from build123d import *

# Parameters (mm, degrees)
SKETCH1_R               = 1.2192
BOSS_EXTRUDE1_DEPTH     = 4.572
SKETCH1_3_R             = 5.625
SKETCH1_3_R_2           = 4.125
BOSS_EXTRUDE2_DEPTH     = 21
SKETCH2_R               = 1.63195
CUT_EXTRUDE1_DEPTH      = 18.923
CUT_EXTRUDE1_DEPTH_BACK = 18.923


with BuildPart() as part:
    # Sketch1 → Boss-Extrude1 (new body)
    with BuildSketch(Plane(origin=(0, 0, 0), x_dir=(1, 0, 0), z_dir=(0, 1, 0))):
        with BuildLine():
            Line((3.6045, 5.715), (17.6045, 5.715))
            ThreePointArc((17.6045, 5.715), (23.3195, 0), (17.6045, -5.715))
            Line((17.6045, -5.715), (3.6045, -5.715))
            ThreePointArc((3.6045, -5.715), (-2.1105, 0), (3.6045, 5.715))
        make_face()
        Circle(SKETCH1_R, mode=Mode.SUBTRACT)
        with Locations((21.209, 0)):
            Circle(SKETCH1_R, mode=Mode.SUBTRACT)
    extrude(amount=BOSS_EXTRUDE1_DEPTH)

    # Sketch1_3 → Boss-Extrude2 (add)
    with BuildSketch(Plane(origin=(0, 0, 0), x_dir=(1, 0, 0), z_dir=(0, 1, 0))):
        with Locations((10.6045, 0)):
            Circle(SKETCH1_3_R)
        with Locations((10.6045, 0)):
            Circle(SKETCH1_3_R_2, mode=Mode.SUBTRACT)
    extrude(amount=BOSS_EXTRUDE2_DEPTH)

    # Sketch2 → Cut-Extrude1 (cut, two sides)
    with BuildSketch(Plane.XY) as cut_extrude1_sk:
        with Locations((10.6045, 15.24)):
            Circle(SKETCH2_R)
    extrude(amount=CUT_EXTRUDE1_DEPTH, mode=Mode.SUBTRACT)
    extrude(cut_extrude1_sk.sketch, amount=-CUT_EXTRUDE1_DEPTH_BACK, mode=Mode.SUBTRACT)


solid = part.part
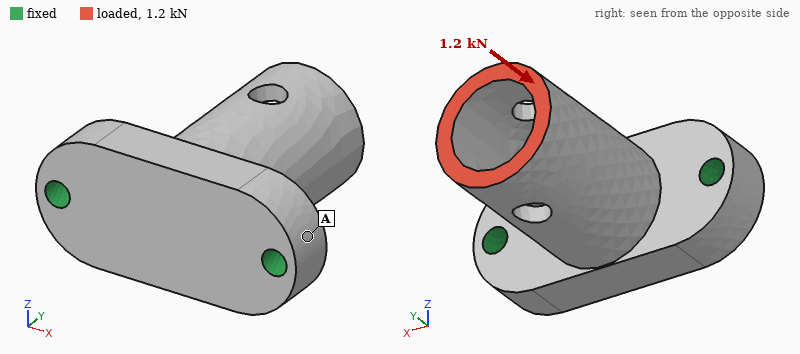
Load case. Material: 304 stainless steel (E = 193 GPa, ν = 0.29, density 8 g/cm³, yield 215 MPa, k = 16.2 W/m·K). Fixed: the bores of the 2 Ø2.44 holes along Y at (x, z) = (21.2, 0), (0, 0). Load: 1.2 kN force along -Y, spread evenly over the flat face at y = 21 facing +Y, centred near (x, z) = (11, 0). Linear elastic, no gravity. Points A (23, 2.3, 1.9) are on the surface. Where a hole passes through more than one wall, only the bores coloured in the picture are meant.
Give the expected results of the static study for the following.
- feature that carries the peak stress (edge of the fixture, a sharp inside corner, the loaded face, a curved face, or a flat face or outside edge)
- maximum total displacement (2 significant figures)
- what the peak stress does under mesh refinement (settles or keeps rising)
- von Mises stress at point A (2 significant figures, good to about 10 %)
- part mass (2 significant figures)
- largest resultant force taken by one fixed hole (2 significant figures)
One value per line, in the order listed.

edge of the fixture
6.1 µm
keeps rising
18 MPa
15 g
610 N
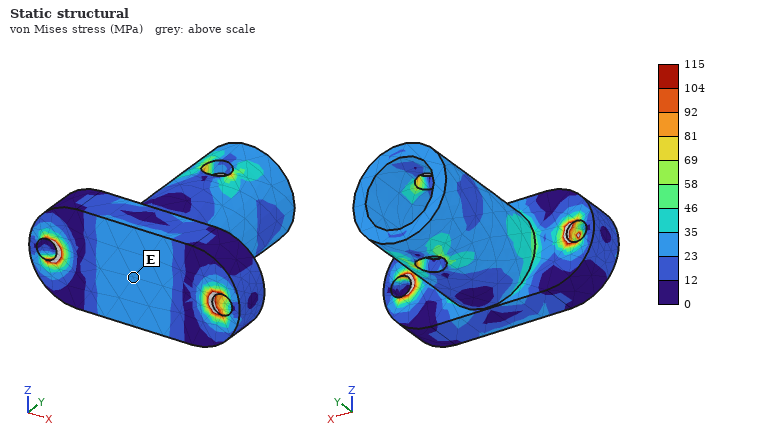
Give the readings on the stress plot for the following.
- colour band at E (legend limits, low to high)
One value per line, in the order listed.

23 to 35 MPa
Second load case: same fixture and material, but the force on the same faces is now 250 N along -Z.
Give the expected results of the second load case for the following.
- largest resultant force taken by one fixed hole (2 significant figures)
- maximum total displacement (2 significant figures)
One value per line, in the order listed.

130 N
24 µm
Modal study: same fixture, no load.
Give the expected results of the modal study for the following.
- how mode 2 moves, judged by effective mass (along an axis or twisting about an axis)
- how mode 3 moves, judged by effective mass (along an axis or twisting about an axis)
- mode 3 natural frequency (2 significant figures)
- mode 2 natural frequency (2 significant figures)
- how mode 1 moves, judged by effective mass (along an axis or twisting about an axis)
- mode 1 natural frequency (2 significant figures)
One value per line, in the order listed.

along X
along Y
28 kHz
18 kHz
along Z
11 kHz
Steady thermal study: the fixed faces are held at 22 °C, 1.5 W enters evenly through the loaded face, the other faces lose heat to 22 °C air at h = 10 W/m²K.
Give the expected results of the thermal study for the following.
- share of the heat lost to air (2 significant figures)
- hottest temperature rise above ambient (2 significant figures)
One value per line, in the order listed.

17 %
40 K
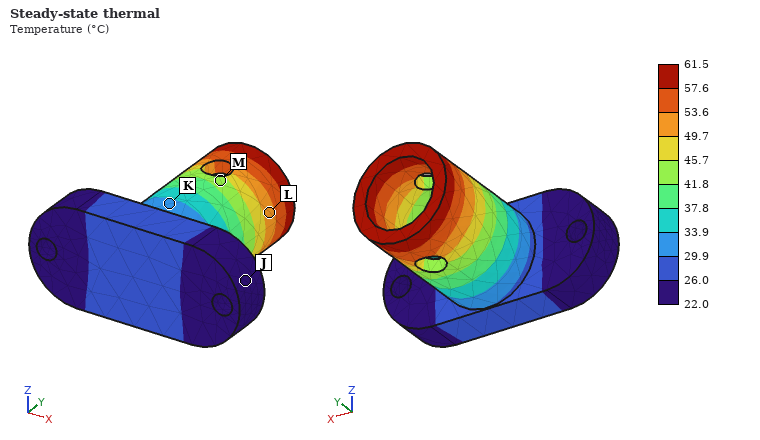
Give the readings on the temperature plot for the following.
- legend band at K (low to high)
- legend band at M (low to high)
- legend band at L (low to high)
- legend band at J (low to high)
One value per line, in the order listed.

29.9 to 33.9 °C
41.8 to 45.7 °C
49.7 to 53.6 °C
22.0 to 26.0 °C
